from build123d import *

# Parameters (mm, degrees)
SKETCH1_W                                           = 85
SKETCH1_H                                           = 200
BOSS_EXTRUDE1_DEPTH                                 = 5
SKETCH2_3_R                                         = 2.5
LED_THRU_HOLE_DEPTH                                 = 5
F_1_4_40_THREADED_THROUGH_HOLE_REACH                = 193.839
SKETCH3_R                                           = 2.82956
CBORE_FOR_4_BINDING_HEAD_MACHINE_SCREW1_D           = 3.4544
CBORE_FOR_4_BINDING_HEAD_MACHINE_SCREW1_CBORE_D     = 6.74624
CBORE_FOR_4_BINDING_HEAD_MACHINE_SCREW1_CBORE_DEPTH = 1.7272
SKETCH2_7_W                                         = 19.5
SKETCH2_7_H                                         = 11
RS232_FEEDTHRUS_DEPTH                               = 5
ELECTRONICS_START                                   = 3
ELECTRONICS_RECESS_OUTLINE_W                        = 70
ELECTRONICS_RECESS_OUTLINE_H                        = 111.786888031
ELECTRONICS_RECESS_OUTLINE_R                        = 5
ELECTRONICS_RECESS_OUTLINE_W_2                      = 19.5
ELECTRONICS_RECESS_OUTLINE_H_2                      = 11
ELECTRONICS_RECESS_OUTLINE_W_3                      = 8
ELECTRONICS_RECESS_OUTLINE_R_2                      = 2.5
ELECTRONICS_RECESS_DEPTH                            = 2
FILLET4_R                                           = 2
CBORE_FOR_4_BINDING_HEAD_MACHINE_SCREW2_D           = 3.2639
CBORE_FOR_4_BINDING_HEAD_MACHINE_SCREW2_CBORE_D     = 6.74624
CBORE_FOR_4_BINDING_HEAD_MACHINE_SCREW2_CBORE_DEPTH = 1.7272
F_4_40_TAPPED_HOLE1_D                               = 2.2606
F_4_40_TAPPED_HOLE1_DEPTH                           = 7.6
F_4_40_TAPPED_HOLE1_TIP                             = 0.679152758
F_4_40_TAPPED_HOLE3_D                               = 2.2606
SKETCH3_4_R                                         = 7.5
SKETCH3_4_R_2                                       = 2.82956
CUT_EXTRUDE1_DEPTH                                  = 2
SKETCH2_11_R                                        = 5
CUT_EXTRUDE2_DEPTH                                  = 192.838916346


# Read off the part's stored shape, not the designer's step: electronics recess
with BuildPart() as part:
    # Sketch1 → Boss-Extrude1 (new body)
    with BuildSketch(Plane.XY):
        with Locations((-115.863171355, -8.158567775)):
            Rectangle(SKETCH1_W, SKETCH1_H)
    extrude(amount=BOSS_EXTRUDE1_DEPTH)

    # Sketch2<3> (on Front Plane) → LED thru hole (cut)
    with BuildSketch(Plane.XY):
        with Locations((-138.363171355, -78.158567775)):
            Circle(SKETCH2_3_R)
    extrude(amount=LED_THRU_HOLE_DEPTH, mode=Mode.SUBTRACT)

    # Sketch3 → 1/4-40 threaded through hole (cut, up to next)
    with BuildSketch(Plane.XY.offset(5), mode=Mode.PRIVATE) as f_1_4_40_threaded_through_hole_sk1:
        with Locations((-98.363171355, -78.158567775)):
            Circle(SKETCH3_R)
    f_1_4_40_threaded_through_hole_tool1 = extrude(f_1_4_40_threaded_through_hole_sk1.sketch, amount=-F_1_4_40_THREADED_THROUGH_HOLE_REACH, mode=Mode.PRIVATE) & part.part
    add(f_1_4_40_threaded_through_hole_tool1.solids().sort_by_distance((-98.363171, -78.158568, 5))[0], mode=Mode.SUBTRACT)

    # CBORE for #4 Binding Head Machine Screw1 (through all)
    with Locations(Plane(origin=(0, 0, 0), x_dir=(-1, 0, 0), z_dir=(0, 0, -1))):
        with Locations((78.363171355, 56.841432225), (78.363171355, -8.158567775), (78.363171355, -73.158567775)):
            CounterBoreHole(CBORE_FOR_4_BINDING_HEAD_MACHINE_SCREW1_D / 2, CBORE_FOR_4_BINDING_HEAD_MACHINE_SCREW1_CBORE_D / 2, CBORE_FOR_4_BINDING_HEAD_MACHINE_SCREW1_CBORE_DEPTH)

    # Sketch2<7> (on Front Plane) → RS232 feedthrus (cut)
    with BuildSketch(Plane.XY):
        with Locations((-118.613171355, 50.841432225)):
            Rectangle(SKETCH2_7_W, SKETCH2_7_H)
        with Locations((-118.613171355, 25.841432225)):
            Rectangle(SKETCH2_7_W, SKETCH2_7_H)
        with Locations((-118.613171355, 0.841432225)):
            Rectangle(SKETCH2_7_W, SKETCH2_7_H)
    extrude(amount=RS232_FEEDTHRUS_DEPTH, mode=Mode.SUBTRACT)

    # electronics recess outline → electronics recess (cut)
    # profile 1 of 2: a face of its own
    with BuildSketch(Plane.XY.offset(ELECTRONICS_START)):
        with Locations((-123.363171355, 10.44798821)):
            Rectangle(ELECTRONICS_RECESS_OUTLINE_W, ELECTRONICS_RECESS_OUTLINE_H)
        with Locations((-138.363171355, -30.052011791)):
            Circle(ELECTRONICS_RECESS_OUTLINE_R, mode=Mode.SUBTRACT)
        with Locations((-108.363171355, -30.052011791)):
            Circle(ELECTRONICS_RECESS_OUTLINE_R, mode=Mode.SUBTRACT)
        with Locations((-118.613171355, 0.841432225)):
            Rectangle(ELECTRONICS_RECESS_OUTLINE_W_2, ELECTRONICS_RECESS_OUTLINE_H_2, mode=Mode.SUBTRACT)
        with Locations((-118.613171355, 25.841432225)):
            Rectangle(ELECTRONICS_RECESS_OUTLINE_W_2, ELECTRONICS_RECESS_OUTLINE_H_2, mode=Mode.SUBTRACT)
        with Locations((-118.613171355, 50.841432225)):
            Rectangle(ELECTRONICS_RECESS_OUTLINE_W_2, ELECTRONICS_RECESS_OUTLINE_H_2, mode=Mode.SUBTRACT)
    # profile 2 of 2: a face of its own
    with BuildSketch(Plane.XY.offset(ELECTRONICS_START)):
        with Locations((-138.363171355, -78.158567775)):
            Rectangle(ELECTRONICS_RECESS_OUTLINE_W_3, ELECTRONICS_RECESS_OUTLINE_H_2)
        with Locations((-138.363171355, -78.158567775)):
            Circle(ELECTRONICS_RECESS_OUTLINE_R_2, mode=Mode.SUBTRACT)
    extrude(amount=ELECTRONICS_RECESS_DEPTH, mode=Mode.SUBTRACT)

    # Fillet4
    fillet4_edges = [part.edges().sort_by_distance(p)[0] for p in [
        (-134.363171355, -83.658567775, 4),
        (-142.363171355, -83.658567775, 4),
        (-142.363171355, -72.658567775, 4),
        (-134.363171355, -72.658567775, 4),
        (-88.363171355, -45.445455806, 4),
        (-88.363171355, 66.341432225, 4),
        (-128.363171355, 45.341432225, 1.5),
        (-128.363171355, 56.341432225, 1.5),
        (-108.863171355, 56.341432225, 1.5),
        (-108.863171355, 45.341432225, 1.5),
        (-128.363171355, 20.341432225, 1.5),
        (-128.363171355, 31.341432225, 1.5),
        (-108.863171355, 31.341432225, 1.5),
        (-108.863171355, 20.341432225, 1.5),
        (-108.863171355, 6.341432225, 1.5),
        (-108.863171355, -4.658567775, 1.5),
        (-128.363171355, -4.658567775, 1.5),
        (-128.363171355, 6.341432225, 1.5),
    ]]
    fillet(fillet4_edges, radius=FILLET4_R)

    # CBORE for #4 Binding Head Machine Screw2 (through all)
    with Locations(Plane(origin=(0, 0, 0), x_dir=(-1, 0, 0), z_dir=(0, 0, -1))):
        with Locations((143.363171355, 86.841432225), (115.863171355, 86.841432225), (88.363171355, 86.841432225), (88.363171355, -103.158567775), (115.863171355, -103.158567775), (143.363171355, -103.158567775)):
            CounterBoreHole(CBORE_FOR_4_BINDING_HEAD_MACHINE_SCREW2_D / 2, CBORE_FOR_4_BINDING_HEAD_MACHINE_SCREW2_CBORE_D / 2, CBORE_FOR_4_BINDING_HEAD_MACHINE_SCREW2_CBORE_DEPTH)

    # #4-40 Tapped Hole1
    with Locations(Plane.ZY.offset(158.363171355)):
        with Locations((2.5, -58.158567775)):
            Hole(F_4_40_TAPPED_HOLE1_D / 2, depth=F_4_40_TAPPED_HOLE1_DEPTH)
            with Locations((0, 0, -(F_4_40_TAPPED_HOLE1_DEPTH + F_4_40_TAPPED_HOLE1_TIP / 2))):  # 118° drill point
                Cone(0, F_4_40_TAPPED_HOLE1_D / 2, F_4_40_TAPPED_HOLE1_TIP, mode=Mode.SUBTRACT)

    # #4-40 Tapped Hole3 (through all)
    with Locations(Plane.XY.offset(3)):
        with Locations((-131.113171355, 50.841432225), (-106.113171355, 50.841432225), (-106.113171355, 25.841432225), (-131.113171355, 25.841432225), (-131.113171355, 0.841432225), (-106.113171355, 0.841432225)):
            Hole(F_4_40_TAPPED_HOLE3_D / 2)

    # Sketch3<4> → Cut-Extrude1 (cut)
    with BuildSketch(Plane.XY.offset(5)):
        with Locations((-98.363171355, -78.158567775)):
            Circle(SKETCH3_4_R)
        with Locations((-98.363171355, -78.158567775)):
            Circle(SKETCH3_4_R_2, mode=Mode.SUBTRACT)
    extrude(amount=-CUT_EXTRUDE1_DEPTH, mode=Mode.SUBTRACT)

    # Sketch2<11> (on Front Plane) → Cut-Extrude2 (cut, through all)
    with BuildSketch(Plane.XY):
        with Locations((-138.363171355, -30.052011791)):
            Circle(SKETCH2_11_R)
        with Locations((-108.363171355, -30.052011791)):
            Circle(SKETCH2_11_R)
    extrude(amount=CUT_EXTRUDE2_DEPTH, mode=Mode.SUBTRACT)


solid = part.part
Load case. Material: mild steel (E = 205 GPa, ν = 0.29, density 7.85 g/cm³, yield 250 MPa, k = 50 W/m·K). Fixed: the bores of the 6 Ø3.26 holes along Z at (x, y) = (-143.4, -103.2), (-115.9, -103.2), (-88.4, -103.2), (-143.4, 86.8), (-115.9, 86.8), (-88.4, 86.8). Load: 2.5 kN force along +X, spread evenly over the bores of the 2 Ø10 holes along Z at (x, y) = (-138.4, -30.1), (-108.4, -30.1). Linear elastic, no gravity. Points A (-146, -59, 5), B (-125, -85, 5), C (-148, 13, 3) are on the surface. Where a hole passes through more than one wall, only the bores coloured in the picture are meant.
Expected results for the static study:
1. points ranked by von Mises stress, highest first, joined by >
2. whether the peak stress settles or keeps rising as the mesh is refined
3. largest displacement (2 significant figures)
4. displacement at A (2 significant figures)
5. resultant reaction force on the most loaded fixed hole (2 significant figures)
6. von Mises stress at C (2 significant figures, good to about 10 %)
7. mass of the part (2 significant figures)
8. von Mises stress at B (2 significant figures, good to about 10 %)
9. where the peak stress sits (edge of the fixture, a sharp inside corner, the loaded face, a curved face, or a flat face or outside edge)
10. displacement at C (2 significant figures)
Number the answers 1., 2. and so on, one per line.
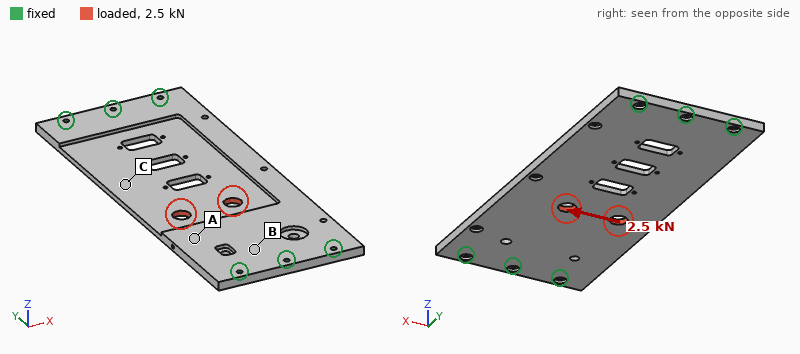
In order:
1. B > C > A
2. keeps rising
3. 18 µm
4. 8.8 µm
5. 1.3 kN
6. 6.0 MPa
7. 510 g
8. 11 MPa
9. edge of the fixture
10. 11 µm
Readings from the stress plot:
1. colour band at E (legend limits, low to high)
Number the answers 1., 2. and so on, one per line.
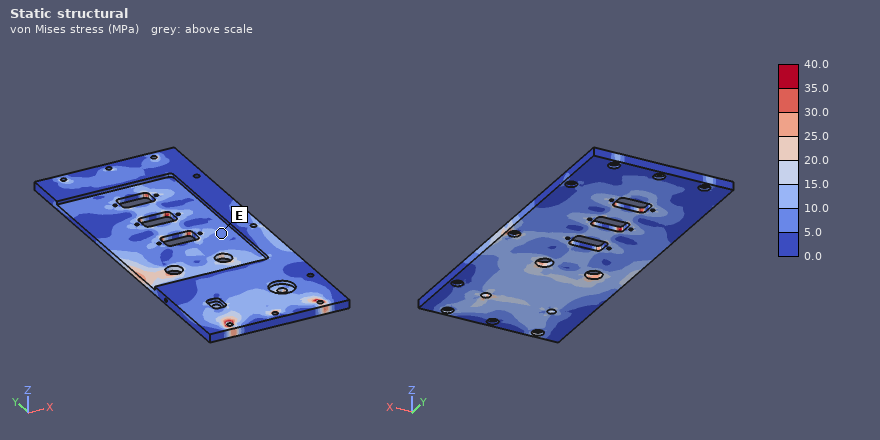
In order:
1. 5.0 to 10.0 MPa
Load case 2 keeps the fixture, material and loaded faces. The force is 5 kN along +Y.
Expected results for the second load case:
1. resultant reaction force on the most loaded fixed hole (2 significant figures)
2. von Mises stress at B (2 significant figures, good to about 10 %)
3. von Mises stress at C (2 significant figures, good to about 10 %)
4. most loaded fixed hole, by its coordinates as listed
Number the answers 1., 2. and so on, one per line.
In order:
1. 1.3 kN
2. 7.8 MPa
3. 9.3 MPa
4. (-143.4, -103.2)
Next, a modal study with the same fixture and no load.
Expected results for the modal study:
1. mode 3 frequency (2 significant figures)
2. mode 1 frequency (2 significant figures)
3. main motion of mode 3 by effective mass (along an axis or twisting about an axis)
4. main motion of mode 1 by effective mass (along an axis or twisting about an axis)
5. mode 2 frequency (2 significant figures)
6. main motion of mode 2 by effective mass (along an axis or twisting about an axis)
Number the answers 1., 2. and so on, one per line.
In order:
1. 1500 Hz
2. 610 Hz
3. twisting about X
4. along Z
5. 1000 Hz
6. twisting about Y
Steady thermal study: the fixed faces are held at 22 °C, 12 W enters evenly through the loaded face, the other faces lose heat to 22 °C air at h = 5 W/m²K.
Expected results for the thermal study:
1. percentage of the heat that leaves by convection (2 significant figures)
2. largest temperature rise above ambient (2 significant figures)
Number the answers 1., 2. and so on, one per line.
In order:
1. 21 %
2. 38 K
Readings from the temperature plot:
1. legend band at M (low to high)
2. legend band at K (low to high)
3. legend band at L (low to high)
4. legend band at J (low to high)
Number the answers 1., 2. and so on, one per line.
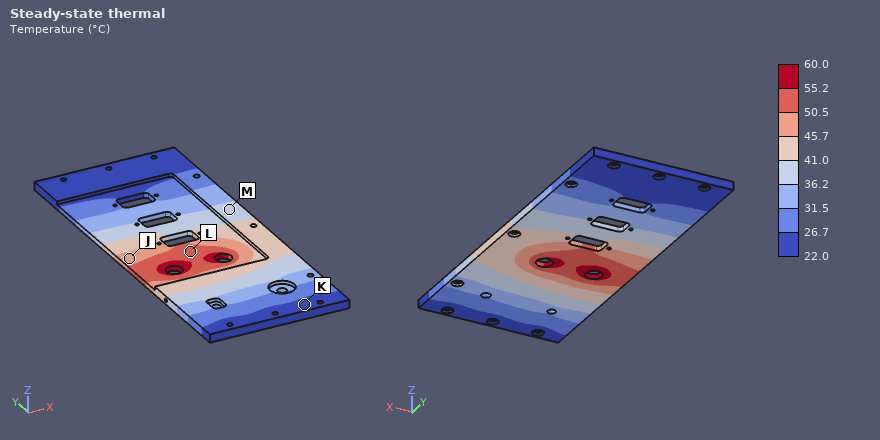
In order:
1. 36.2 to 41.0 °C
2. 22.0 to 26.7 °C
3. 50.5 to 55.2 °C
4. 45.7 to 50.5 °C
